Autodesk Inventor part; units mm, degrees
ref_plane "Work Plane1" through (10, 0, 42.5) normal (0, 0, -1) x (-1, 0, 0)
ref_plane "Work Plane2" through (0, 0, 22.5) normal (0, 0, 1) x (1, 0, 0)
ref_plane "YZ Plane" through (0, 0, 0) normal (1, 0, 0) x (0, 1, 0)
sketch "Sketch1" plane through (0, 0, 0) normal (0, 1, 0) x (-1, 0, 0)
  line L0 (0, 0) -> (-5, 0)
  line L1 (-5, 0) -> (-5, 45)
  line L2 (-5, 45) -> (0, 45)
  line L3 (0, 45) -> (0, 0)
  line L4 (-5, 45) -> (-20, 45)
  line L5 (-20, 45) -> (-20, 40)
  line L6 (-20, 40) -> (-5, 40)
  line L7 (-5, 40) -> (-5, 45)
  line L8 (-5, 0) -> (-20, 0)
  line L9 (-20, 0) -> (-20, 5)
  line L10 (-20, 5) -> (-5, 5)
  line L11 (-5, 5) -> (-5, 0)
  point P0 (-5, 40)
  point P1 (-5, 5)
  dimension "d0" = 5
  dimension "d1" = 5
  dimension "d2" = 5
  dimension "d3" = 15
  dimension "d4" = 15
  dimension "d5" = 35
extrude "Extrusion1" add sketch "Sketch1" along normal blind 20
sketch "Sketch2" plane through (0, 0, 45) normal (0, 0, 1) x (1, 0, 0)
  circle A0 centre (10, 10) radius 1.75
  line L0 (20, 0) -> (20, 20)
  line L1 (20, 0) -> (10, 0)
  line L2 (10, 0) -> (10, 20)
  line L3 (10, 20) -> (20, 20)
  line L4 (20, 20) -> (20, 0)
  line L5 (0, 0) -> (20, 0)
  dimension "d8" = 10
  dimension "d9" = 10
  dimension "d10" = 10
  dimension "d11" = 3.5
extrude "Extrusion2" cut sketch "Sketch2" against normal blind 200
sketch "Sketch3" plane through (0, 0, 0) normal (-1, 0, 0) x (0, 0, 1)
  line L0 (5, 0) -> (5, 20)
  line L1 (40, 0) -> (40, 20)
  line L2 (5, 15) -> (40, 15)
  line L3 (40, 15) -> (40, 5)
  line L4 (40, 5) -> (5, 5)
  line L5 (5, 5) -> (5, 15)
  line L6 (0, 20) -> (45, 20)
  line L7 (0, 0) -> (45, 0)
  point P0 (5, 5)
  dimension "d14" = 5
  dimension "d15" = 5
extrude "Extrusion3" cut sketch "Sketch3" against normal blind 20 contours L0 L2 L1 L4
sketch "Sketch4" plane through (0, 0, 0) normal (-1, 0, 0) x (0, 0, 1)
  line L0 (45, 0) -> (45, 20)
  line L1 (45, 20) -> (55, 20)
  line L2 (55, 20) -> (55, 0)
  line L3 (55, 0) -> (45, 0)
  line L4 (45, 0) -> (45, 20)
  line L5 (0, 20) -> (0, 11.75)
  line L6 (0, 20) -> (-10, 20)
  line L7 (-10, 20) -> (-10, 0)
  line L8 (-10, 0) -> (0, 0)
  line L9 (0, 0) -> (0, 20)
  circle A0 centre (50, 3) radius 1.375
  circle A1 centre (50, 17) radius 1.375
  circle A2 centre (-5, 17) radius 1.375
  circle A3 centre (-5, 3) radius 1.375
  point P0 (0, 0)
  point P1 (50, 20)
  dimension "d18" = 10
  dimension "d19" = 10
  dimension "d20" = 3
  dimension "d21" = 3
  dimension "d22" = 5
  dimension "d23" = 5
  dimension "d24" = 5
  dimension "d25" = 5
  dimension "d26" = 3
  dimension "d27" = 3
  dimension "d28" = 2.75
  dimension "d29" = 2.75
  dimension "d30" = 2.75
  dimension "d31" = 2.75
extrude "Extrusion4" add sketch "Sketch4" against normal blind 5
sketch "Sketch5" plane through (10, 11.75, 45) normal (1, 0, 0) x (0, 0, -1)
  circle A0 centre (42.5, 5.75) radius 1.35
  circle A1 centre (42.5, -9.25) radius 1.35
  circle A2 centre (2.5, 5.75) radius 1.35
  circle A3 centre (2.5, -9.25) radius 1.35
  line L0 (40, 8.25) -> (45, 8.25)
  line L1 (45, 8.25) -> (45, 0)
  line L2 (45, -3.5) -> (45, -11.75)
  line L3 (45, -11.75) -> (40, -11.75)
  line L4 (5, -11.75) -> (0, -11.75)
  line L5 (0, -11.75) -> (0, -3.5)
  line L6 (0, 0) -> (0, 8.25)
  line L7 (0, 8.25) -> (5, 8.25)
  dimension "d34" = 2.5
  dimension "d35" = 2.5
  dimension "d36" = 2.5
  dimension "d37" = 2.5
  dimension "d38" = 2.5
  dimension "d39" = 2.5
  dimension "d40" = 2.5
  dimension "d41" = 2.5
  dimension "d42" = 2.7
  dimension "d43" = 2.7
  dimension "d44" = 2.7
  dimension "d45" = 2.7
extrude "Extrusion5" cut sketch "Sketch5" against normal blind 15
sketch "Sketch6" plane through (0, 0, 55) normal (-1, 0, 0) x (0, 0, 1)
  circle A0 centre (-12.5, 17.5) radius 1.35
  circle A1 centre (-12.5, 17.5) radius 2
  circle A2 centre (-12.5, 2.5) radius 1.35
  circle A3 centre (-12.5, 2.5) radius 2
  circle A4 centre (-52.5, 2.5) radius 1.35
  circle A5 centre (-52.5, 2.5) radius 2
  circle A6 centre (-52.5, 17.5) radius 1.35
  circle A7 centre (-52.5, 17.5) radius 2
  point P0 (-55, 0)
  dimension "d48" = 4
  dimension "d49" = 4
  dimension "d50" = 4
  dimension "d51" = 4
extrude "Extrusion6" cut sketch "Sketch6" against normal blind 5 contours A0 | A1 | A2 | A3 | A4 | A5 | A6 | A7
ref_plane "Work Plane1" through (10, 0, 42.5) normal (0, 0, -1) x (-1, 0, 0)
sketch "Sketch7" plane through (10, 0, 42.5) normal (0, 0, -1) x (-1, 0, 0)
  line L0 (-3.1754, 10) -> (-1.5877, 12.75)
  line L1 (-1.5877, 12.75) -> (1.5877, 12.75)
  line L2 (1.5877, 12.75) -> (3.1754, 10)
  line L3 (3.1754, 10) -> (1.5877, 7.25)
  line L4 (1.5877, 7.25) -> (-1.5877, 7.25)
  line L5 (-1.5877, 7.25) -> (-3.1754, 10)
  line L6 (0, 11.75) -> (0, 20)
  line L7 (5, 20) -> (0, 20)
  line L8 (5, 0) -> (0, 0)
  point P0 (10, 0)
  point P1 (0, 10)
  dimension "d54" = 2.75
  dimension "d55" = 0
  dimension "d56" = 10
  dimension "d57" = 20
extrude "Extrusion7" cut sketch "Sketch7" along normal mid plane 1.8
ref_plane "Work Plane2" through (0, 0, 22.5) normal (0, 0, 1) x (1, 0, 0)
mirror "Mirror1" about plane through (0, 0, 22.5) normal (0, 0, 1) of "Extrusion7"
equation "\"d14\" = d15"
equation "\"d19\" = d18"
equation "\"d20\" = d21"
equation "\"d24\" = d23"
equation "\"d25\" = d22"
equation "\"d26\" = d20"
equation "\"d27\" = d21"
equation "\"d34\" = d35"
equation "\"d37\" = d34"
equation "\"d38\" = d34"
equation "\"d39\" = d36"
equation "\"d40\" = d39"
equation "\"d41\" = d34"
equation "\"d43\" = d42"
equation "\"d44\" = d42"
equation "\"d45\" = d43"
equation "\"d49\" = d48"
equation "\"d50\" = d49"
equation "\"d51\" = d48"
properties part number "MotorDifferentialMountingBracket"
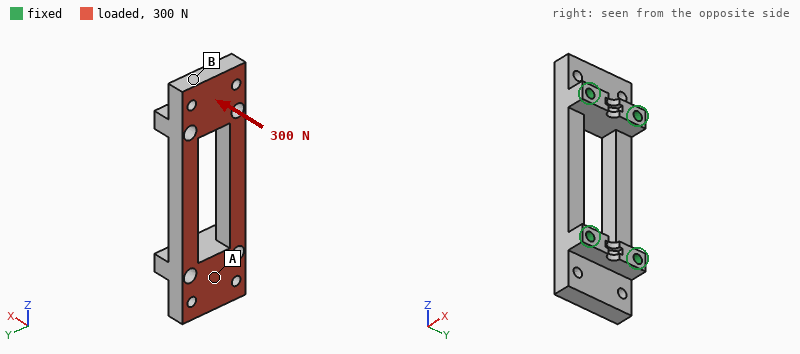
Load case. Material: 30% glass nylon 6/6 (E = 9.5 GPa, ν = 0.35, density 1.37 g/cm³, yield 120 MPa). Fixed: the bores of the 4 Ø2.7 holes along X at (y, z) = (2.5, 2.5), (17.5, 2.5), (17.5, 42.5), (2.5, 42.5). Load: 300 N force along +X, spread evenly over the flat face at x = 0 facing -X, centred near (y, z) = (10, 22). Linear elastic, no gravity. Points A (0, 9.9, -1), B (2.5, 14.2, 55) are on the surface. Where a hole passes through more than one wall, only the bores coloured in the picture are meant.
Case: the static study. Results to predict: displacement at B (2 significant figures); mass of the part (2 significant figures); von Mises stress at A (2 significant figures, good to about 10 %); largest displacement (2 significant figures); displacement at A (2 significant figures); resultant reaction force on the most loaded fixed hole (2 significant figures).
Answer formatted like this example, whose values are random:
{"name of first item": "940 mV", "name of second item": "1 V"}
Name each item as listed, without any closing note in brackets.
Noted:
{"displacement at B": "16 µm", "mass of the part": "7.1 g", "von Mises stress at A": "3.0 MPa", "largest displacement": "26 µm", "displacement at A": "5.8 µm", "resultant reaction force on the most loaded fixed hole": "78 N"}
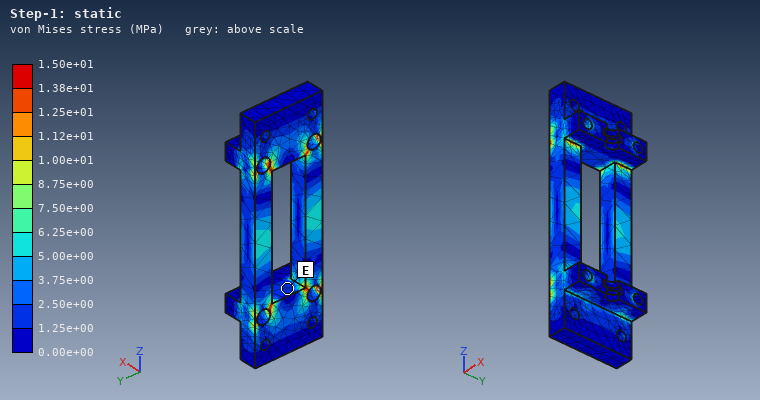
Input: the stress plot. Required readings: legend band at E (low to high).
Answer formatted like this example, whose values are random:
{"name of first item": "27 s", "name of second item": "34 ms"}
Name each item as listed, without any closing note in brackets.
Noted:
{"legend band at E": "1.25e+00 to 2.50e+00 MPa"}
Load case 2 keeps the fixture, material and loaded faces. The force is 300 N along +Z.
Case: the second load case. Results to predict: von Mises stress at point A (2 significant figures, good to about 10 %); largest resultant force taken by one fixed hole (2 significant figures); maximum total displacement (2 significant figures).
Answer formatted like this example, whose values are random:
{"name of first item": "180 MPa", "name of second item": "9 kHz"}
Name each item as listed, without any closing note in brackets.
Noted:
{"von Mises stress at point A": "2.7 MPa", "largest resultant force taken by one fixed hole": "76 N", "maximum total displacement": "33 µm"}
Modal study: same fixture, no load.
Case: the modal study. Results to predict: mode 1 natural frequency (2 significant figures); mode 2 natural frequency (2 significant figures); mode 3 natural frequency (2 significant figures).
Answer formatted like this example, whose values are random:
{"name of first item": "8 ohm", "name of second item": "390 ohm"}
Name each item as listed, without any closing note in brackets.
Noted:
{"mode 1 natural frequency": "6600 Hz", "mode 2 natural frequency": "7200 Hz", "mode 3 natural frequency": "7300 Hz"}
